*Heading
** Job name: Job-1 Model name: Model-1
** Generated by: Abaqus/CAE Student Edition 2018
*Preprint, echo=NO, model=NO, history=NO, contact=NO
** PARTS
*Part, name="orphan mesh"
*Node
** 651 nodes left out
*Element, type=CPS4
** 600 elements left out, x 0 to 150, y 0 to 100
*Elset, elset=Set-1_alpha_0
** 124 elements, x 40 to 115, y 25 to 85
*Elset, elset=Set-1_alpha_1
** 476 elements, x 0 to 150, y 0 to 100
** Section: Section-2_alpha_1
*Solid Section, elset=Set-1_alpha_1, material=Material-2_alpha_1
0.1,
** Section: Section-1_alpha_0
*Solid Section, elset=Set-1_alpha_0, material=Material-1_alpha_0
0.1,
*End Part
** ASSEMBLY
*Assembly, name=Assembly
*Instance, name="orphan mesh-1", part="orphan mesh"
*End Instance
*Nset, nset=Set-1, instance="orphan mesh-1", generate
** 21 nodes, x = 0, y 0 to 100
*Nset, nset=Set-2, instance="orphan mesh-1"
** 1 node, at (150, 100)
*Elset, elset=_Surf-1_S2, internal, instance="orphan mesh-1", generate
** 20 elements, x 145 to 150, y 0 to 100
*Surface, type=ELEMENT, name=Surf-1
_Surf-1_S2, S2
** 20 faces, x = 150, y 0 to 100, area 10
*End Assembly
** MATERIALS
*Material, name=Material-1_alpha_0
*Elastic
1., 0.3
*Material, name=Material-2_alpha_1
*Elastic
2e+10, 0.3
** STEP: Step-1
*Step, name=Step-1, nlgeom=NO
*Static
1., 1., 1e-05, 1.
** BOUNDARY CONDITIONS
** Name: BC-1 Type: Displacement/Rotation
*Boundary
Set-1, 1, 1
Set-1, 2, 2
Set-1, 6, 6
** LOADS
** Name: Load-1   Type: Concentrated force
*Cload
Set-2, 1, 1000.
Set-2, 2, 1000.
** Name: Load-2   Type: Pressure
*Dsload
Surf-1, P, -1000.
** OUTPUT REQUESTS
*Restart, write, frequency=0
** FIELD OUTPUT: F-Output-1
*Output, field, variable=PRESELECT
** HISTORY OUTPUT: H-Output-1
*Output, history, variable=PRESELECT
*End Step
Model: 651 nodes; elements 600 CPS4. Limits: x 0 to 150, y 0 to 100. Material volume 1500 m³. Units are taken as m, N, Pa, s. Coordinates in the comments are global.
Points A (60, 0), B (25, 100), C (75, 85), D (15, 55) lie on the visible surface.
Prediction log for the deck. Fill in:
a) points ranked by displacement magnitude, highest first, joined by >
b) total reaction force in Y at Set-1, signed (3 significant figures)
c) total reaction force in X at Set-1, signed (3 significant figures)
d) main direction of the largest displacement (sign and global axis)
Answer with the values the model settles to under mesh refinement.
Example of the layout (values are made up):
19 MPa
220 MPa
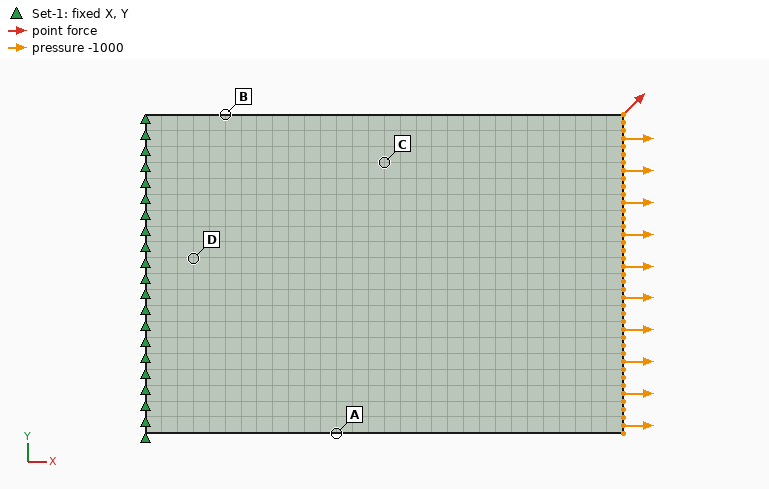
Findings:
A > C > B > D
-1000 N
-11000 N
+X
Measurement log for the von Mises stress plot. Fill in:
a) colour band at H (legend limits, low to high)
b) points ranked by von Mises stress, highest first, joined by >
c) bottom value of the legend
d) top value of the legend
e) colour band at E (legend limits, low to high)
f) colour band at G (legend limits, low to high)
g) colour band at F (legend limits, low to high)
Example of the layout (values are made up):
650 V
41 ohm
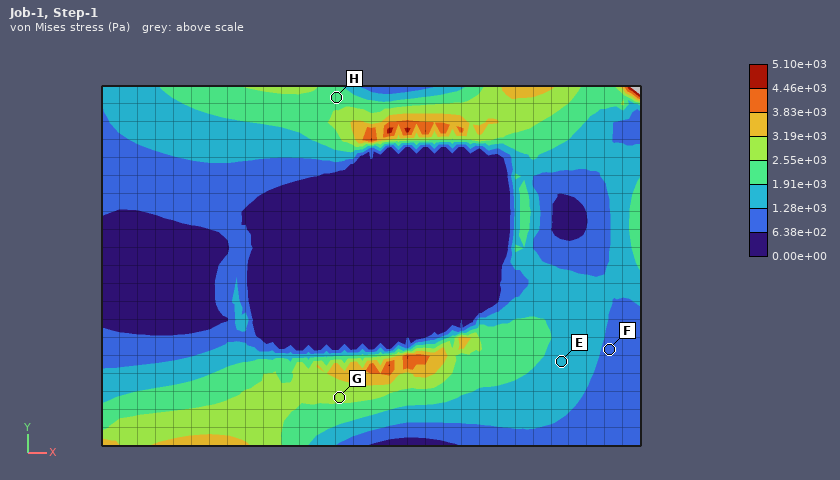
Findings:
1.91e+03 to 2.55e+03 Pa
G > H > E > F
0.00e+00 Pa
5.10e+03 Pa
1.28e+03 to 1.91e+03 Pa
2.55e+03 to 3.19e+03 Pa
6.38e+02 to 1.28e+03 Pa
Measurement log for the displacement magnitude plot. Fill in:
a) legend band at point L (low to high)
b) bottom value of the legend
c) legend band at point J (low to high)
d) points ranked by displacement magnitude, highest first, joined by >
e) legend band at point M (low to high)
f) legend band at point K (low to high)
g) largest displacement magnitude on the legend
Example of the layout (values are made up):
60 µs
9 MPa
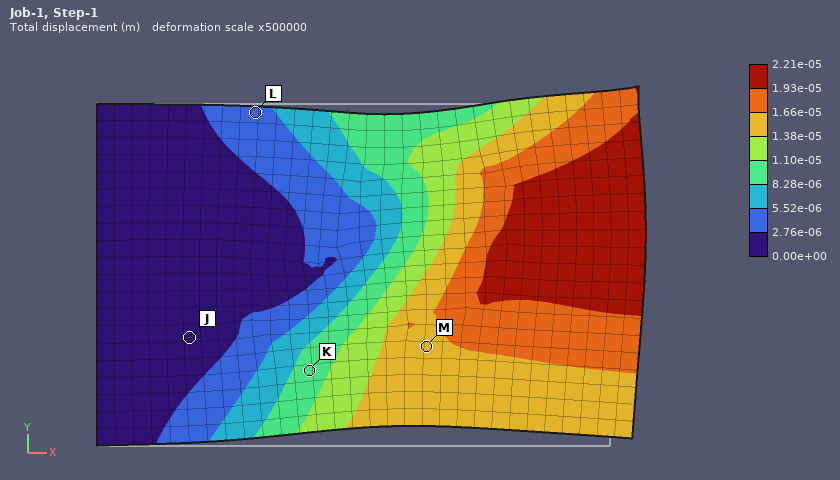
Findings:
2.76e-06 to 5.52e-06 m
0.00e+00 m
0.00e+00 to 2.76e-06 m
M > K > L > J
1.38e-05 to 1.66e-05 m
8.28e-06 to 1.10e-05 m
2.21e-05 m
